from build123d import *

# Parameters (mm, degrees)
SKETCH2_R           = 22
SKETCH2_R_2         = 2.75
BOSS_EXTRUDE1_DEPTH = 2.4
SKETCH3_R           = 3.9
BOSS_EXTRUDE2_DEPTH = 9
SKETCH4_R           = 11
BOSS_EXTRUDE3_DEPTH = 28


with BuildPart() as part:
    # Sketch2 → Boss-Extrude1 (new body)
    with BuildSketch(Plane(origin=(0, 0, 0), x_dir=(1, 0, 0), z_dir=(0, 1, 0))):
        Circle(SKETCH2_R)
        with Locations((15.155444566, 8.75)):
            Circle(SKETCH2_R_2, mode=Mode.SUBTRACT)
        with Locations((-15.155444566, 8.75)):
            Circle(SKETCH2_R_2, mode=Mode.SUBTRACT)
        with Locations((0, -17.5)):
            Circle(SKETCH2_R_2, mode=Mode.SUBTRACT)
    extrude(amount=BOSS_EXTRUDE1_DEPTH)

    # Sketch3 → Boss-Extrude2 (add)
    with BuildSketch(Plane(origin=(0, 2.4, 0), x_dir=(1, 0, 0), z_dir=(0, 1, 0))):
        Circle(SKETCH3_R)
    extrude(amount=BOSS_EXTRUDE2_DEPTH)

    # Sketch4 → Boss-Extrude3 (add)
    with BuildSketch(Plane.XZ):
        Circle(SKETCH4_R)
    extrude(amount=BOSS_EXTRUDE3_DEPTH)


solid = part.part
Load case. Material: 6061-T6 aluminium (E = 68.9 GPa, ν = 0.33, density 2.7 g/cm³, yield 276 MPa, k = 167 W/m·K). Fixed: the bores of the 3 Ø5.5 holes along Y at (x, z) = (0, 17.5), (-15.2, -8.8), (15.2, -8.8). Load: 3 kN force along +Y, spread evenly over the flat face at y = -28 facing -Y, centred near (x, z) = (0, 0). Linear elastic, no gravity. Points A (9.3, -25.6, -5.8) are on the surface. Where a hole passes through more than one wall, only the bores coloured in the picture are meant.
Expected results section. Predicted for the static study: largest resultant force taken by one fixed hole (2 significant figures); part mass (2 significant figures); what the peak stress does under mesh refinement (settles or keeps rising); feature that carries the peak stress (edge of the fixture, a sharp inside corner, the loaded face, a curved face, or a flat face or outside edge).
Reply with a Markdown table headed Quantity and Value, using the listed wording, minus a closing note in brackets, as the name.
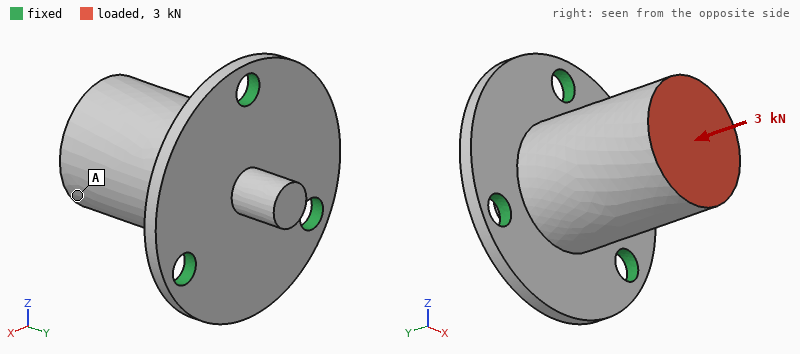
| Quantity | Value |
|---|---|
| largest resultant force taken by one fixed hole | 1.1 kN |
| part mass | 39 g |
| what the peak stress does under mesh refinement | keeps rising |
| feature that carries the peak stress | edge of the fixture |
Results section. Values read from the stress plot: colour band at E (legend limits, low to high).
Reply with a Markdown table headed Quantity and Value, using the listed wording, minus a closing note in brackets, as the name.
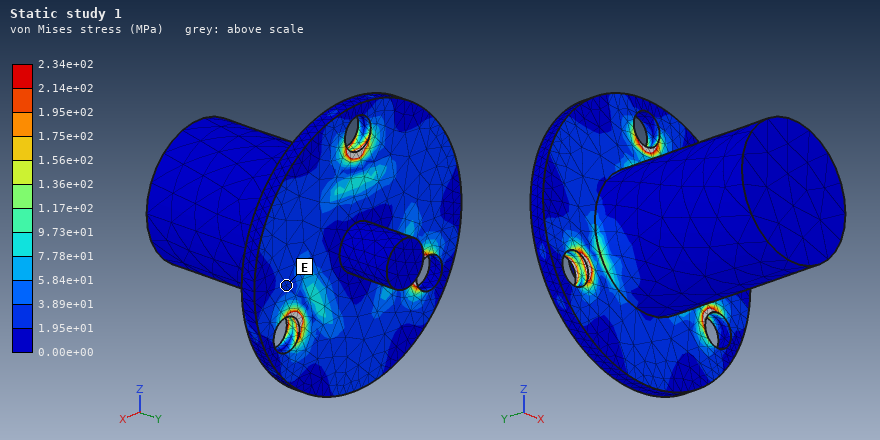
| Quantity | Value |
|---|---|
| colour band at E | 1.95e+01 to 3.89e+01 MPa |
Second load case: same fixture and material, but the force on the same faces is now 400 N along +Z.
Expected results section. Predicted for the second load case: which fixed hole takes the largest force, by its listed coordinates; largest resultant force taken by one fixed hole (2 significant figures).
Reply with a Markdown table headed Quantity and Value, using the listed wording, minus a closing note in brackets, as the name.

| Quantity | Value |
|---|---|
| which fixed hole takes the largest force, by its listed coordinates | (0, 17.5) |
| largest resultant force taken by one fixed hole | 580 N |
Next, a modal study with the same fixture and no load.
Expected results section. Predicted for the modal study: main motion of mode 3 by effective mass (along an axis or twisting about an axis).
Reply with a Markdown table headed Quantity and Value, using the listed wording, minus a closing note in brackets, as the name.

| Quantity | Value |
|---|---|
| main motion of mode 3 by effective mass | along Y |
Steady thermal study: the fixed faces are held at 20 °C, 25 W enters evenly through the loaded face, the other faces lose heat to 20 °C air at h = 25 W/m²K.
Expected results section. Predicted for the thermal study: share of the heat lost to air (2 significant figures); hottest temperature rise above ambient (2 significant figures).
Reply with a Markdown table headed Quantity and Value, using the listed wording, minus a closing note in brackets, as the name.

| Quantity | Value |
|---|---|
| share of the heat lost to air | 4.2 % |
| hottest temperature rise above ambient | 20 K |
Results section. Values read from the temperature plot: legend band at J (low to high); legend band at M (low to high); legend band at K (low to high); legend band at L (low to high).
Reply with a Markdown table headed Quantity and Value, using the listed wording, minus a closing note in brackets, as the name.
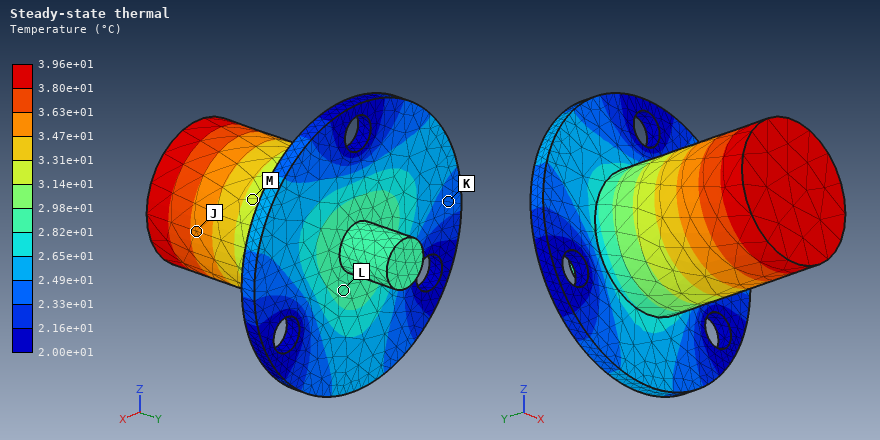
| Quantity | Value |
|---|---|
| legend band at J | 3.47e+01 to 3.63e+01 °C |
| legend band at M | 3.14e+01 to 3.31e+01 °C |
| legend band at K | 2.33e+01 to 2.49e+01 °C |
| legend band at L | 2.82e+01 to 2.98e+01 °C |
